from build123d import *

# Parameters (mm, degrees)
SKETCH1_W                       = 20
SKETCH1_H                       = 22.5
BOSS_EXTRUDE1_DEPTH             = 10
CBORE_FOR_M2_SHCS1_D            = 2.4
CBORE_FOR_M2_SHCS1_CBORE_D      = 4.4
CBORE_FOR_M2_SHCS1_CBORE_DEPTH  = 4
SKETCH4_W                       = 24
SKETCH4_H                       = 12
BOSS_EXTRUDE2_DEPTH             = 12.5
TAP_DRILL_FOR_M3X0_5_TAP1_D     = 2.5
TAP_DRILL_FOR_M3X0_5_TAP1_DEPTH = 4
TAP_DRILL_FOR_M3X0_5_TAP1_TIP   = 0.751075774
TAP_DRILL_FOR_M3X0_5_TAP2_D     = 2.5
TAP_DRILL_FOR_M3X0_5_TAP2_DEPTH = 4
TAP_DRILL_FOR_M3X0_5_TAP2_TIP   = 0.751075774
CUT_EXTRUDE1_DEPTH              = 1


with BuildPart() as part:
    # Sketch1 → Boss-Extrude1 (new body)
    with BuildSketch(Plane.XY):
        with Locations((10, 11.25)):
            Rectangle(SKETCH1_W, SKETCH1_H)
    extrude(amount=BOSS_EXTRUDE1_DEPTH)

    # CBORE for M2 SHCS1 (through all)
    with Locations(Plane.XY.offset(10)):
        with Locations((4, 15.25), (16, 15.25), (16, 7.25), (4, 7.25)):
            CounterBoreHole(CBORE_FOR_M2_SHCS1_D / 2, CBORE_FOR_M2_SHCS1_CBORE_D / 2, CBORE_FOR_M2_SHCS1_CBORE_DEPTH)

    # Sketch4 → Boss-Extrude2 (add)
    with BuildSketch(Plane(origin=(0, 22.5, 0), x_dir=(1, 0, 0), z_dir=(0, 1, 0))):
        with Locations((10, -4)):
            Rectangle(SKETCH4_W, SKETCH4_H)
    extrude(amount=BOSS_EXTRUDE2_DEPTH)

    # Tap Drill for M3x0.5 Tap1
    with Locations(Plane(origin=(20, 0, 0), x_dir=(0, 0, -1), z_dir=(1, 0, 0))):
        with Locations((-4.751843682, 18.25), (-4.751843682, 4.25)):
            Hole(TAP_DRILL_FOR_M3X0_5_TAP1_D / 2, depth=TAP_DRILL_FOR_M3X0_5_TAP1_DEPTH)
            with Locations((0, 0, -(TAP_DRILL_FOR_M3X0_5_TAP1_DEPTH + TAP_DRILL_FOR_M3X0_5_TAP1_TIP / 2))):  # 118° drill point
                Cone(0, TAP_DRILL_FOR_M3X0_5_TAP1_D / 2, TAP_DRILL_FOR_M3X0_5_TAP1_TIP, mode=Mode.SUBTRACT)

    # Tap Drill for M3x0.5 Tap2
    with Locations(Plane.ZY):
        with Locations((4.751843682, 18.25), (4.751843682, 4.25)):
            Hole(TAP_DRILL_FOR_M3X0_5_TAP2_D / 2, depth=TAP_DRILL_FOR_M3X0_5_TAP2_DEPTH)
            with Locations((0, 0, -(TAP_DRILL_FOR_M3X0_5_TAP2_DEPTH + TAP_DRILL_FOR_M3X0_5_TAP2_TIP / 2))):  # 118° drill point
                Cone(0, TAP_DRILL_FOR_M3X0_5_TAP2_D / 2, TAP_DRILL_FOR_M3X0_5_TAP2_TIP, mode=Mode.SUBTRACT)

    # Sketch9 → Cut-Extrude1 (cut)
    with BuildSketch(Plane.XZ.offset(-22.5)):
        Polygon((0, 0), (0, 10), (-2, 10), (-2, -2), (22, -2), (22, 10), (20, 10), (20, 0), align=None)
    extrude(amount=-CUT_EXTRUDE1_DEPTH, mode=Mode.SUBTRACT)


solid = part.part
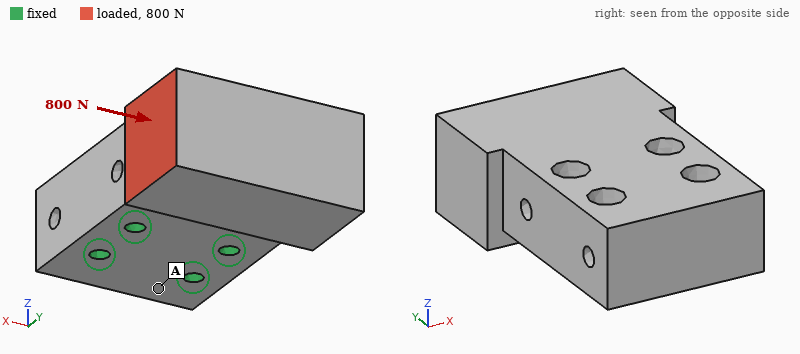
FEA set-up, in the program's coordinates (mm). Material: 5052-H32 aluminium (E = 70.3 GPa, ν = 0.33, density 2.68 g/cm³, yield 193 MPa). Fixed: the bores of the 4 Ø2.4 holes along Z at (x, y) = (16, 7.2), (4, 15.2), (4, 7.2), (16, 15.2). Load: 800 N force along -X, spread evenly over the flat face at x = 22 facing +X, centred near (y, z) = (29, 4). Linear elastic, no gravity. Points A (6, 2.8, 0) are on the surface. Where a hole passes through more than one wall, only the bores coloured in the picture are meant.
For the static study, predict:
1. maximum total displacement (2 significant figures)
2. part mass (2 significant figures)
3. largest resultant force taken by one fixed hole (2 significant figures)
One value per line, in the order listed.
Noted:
9.3 µm
20 g
770 N
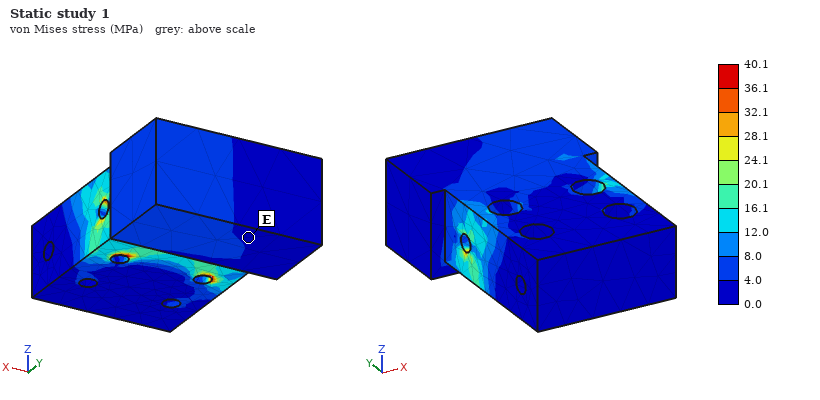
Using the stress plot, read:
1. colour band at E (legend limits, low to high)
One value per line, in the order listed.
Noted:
0.0 to 4.0 MPa
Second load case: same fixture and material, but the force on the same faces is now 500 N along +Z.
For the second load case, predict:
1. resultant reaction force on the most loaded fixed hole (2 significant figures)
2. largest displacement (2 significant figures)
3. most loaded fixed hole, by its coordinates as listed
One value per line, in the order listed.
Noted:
810 N
23 µm
(16, 15.2)
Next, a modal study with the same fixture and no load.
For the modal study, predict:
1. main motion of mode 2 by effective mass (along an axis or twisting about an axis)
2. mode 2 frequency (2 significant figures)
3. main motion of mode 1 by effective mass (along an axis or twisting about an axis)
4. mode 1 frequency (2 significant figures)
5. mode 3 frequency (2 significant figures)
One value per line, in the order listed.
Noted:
along X
18 kHz
along Z
11 kHz
22 kHz
